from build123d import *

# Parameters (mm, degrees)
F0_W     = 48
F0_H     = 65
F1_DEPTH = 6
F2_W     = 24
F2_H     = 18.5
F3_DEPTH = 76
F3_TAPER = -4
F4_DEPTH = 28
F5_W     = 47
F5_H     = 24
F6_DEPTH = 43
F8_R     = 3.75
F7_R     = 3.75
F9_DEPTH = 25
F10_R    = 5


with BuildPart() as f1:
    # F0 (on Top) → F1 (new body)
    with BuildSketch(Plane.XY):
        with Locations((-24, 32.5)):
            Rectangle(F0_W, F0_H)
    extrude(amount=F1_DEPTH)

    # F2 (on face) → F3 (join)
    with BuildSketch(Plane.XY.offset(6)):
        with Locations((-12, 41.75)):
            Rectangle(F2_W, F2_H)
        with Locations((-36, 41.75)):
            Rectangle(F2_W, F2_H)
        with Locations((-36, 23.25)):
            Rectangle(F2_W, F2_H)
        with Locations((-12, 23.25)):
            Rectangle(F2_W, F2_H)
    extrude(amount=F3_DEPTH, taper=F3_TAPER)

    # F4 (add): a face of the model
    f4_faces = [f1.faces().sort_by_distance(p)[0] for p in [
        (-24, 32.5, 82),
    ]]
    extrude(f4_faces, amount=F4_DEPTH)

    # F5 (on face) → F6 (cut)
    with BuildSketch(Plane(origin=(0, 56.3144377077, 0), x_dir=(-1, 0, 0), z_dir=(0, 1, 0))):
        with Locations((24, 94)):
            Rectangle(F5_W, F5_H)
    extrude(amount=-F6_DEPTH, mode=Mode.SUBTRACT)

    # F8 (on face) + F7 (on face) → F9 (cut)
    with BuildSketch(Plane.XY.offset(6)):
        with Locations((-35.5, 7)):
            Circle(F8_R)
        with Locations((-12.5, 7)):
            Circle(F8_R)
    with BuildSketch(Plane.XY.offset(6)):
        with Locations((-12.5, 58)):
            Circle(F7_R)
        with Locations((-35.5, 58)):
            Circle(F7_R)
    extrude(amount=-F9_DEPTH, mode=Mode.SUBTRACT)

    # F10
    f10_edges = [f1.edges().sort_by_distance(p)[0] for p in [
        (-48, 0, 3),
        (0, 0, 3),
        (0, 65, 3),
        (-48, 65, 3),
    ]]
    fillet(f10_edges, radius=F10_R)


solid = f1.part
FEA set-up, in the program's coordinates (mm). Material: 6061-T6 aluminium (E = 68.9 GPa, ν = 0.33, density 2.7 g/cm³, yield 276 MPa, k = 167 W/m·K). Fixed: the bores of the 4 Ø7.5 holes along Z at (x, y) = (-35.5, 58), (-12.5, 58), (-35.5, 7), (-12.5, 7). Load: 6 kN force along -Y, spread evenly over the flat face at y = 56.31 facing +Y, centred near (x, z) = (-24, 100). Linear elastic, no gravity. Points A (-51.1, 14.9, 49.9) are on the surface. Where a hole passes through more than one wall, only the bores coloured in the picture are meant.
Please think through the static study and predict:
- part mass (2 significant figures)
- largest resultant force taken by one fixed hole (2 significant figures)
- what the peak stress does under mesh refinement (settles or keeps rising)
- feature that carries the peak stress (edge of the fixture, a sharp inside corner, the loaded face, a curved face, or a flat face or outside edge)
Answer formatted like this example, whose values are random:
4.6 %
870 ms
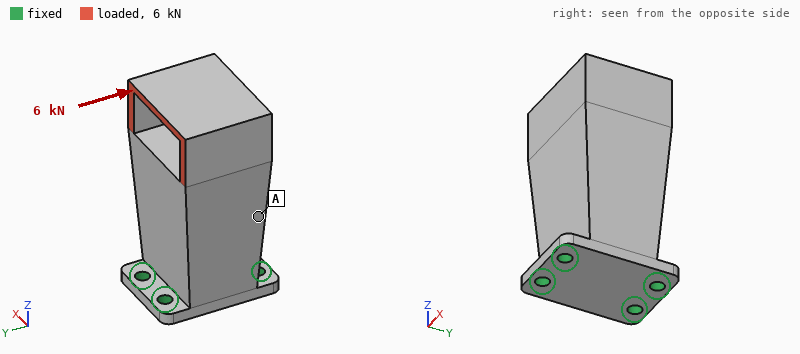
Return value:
590 g
7.2 kN
keeps rising
edge of the fixture
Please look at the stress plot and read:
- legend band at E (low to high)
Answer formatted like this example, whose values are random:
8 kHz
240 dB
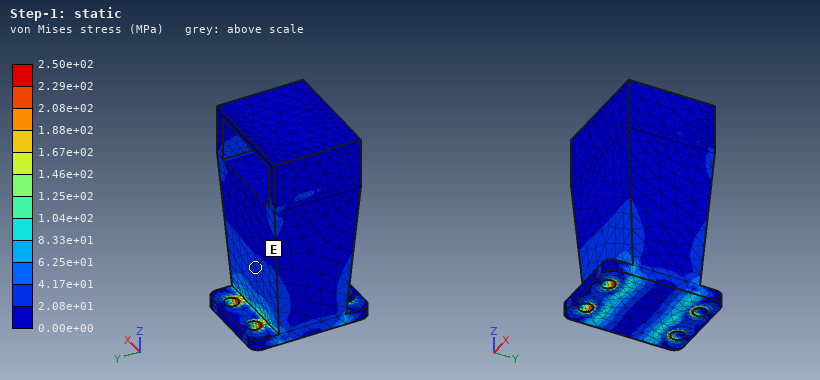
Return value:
2.08e+01 to 4.17e+01 MPa
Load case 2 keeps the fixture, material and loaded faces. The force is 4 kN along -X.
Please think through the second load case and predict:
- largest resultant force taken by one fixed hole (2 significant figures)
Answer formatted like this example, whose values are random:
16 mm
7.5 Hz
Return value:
7.7 kN
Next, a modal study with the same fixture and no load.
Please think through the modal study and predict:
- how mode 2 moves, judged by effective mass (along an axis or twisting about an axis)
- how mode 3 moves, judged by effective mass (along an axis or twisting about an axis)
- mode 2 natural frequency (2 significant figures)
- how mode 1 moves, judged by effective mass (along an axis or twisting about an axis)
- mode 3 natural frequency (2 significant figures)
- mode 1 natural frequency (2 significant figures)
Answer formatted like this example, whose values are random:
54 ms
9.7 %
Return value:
along Y
twisting about Z
1800 Hz
along X
5200 Hz
1200 Hz
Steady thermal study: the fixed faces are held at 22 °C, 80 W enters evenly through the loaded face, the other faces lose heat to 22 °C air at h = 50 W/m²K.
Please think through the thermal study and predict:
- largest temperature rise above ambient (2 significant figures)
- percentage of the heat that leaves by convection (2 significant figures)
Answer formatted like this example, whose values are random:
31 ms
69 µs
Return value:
48 K
35 %
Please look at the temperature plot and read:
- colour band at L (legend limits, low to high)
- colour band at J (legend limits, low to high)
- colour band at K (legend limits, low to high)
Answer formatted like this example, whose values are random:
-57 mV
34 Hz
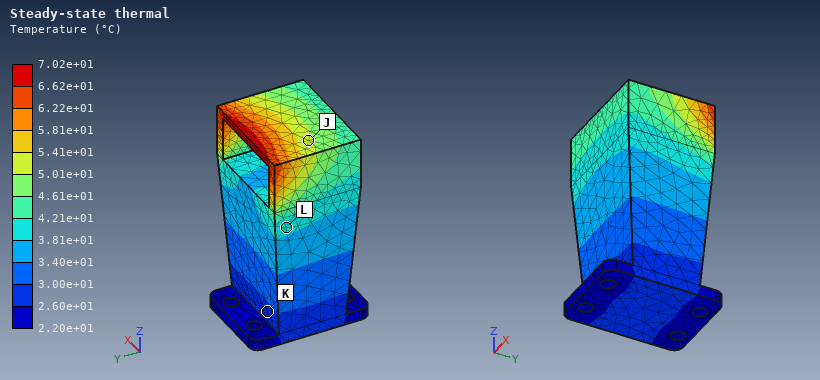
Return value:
3.81e+01 to 4.21e+01 °C
5.01e+01 to 5.41e+01 °C
2.60e+01 to 3.00e+01 °C
